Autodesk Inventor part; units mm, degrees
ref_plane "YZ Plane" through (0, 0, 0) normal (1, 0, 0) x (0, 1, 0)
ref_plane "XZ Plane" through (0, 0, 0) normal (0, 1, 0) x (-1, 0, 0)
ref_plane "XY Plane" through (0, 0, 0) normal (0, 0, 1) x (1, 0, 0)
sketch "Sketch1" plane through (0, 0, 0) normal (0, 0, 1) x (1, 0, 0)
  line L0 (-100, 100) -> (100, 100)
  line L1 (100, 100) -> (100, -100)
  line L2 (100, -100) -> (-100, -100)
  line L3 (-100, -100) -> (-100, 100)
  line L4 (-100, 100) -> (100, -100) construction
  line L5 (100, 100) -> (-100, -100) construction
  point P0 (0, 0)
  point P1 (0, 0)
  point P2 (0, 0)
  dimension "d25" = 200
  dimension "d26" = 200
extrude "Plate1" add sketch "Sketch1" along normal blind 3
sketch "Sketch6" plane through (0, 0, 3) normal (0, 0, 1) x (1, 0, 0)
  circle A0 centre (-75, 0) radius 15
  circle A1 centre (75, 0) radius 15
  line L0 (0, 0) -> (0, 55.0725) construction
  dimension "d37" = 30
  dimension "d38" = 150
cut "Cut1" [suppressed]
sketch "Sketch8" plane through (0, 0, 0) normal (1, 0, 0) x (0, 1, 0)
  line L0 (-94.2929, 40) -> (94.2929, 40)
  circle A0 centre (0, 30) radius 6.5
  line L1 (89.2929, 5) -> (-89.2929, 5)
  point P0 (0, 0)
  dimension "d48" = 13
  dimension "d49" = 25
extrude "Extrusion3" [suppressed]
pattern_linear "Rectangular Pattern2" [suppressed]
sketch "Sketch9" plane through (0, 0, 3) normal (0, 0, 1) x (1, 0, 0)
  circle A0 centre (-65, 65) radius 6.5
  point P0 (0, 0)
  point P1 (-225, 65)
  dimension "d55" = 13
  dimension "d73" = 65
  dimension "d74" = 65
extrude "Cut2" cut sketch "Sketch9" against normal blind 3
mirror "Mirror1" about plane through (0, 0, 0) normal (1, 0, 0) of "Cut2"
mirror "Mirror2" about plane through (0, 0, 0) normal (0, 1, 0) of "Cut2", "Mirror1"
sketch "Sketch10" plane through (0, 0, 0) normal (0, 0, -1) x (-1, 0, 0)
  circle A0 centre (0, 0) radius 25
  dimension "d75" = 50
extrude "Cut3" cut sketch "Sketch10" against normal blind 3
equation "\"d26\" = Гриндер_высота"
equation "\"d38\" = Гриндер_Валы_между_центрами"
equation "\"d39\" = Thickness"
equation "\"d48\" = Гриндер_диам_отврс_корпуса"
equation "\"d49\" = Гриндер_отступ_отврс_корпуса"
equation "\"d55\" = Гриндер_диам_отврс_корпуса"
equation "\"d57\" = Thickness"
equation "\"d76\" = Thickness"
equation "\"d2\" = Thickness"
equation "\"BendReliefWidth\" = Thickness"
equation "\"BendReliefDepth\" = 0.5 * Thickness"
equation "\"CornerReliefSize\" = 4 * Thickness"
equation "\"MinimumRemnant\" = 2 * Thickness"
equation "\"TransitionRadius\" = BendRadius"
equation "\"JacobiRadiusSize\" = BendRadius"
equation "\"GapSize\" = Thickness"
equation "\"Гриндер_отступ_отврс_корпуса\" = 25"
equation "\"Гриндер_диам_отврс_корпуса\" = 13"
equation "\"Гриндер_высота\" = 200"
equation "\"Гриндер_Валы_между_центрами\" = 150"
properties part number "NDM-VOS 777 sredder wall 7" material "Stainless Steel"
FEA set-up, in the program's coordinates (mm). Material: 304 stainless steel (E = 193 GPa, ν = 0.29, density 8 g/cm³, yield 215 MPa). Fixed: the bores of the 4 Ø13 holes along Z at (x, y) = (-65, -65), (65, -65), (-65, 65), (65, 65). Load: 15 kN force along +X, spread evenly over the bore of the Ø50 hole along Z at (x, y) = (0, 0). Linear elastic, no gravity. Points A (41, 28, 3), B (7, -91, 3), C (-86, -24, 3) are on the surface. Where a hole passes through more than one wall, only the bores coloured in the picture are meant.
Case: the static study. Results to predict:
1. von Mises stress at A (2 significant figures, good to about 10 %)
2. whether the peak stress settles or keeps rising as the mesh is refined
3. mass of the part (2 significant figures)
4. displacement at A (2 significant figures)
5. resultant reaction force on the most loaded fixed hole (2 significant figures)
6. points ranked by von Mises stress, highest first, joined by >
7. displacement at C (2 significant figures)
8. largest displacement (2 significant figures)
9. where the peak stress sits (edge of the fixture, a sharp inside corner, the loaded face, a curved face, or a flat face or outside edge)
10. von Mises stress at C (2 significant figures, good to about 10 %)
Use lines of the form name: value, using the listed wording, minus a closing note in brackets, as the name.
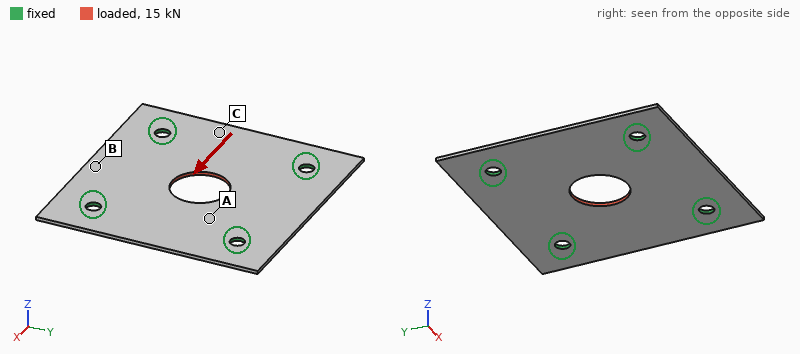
von Mises stress at A: 26 MPa
whether the peak stress settles or keeps rising as the mesh is refined: keeps rising
mass of the part: 900 g
displacement at A: 8.8 µm
resultant reaction force on the most loaded fixed hole: 4.0 kN
points ranked by von Mises stress, highest first, joined by >: A > C > B
displacement at C: 8.0 µm
largest displacement: 14 µm
where the peak stress sits: edge of the fixture
von Mises stress at C: 12 MPa
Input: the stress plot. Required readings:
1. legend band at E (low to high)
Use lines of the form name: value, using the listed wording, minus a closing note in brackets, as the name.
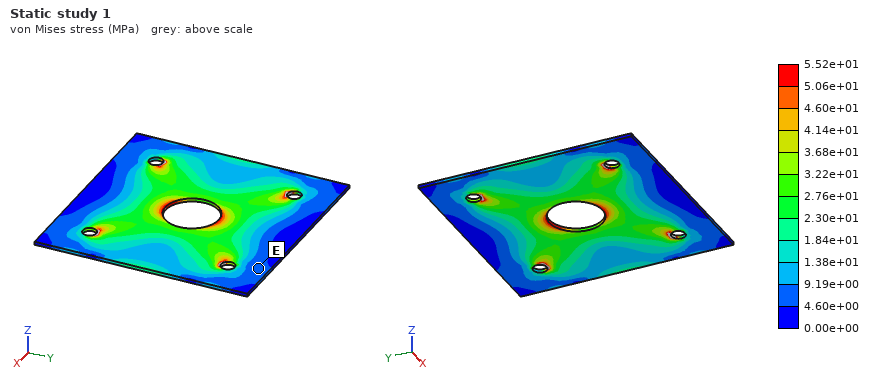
legend band at E: 4.60e+00 to 9.19e+00 MPa
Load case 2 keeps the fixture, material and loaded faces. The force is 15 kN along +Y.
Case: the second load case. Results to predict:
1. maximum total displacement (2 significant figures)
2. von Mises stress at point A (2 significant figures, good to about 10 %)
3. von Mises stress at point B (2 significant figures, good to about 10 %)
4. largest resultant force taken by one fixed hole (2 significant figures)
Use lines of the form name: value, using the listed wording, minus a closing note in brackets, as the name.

maximum total displacement: 14 µm
von Mises stress at point A: 26 MPa
von Mises stress at point B: 15 MPa
largest resultant force taken by one fixed hole: 4.0 kN
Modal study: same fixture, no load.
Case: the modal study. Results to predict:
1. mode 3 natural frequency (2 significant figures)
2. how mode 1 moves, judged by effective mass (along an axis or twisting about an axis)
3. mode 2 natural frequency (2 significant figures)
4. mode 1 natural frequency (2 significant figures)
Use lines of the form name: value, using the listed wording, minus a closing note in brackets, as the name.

mode 3 natural frequency: 960 Hz
how mode 1 moves, judged by effective mass: along Z
mode 2 natural frequency: 930 Hz
mode 1 natural frequency: 750 Hz
